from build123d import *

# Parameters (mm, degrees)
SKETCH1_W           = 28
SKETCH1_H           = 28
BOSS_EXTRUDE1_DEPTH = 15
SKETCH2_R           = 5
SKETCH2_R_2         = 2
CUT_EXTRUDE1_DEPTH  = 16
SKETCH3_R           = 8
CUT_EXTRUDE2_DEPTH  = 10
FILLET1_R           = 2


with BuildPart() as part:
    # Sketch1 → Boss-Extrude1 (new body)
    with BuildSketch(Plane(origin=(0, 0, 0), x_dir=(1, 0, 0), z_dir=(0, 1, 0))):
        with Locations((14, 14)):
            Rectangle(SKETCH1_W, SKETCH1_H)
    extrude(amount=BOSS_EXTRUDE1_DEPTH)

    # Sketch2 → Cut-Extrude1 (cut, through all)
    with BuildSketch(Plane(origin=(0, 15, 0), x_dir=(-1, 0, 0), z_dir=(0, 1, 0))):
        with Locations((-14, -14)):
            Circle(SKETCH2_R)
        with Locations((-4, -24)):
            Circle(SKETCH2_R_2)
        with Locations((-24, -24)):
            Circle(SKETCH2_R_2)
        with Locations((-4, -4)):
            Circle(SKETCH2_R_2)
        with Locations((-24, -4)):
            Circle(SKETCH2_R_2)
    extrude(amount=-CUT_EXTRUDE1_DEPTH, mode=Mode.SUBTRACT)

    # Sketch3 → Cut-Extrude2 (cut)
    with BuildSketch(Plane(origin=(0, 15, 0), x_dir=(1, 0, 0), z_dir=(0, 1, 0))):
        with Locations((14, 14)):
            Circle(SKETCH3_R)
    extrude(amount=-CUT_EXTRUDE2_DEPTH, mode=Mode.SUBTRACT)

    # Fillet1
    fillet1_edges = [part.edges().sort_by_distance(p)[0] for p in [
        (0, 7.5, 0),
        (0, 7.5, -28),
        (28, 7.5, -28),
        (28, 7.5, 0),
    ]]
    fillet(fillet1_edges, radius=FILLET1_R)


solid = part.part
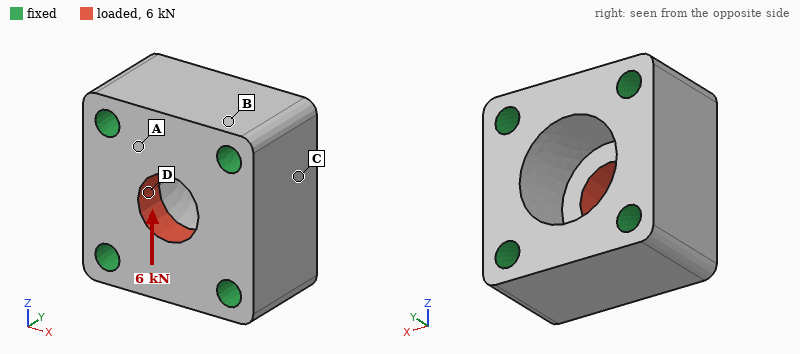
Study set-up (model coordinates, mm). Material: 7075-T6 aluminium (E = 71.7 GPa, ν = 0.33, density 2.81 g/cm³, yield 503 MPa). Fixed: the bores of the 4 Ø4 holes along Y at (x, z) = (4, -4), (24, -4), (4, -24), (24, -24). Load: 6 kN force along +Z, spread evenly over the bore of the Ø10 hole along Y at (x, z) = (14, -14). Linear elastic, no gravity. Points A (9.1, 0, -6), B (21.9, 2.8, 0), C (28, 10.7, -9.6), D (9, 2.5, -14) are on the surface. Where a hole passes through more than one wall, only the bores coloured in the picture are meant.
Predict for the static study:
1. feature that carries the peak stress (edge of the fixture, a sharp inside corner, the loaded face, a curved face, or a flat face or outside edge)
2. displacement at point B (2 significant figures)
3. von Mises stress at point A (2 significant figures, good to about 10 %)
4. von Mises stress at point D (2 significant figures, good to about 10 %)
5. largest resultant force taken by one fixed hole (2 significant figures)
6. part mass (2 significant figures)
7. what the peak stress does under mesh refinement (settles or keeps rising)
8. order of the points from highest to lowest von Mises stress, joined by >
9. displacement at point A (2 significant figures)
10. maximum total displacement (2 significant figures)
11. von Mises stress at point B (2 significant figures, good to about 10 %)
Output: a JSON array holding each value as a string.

["edge of the fixture", "1.2 µm", "39 MPa", "65 MPa", "1.6 kN", "24 g", "keeps rising", "D > A > B > C", "3.4 µm", "7.3 µm", "18 MPa"]
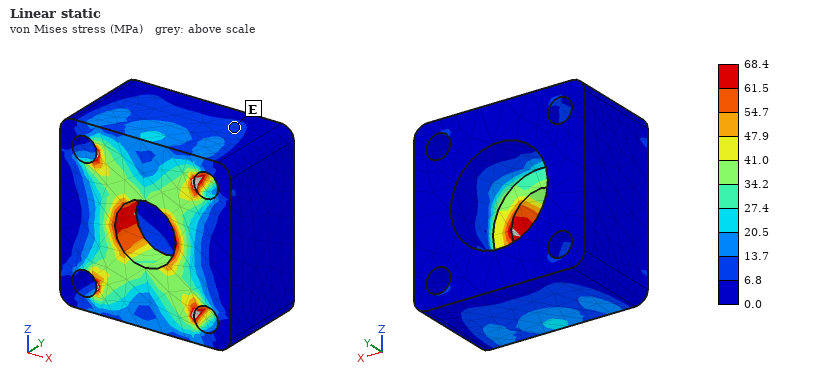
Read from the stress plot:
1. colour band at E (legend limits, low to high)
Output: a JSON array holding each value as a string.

["6.8 to 13.7 MPa"]
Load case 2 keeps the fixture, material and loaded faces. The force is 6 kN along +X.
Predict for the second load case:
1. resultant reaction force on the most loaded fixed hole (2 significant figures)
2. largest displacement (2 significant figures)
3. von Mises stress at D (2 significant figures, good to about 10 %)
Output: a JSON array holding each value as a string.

["1.6 kN", "7.4 µm", "32 MPa"]
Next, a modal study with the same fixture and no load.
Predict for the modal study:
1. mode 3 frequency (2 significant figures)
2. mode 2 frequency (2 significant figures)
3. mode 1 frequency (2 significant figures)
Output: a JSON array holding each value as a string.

["76 kHz", "74 kHz", "61 kHz"]
